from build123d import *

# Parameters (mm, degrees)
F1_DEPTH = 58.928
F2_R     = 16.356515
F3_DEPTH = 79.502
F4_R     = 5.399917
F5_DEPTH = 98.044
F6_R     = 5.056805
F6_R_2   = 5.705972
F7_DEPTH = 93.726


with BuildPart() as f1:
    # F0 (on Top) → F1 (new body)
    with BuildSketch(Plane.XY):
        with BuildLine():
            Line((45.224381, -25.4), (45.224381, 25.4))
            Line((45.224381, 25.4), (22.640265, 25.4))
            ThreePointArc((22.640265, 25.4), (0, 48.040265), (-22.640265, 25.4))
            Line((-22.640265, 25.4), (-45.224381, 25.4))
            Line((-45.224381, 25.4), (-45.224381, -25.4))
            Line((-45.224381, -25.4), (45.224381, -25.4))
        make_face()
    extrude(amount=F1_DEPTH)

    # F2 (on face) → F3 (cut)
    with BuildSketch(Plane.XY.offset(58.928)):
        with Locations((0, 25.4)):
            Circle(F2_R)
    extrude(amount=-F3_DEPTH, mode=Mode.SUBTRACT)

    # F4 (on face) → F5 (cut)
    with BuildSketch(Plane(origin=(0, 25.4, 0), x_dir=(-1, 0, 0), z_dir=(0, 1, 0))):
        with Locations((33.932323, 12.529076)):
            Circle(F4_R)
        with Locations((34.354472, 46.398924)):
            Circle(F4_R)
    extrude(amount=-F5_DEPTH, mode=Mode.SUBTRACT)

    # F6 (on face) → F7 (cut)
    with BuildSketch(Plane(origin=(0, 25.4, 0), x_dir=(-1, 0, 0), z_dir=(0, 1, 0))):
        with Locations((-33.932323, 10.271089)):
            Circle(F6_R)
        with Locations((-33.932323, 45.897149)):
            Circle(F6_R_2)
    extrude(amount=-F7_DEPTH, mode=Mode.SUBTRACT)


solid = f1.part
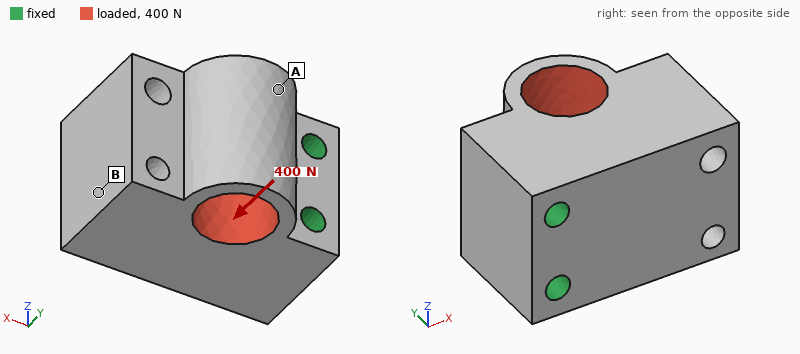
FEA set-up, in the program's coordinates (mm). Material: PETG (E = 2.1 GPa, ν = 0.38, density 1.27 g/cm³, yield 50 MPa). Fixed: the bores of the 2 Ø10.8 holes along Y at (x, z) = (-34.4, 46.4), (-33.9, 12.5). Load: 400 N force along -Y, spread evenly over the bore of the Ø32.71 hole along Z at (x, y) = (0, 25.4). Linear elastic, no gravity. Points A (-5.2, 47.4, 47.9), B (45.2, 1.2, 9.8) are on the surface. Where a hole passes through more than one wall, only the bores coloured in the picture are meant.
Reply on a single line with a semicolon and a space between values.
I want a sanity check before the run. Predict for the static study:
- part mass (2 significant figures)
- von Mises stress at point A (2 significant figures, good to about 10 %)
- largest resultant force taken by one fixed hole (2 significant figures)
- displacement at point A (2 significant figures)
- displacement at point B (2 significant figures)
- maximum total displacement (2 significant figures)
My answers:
320 g; 0.41 MPa; 200 N; 28 µm; 34 µm; 37 µm
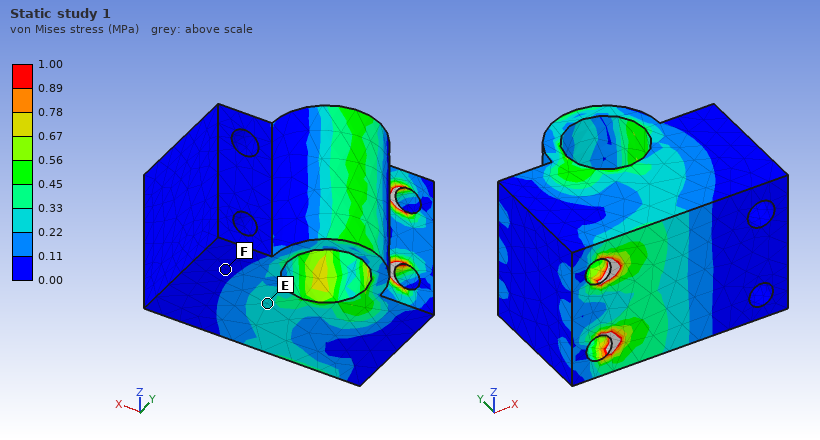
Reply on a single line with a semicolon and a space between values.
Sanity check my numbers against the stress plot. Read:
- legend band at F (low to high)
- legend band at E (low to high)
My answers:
0.00 to 0.11 MPa; 0.22 to 0.33 MPa
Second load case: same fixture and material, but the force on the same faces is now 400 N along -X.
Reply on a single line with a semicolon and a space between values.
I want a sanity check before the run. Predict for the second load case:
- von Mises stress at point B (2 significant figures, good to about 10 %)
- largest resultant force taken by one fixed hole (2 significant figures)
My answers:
0.096 MPa; 200 N
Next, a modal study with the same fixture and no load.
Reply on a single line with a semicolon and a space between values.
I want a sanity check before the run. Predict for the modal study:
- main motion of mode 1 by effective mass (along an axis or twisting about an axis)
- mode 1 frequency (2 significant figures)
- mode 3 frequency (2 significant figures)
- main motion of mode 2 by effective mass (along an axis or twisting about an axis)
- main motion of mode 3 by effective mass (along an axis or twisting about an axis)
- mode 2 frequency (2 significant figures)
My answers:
along Y; 1100 Hz; 2100 Hz; along Z; twisting about X; 1300 Hz
